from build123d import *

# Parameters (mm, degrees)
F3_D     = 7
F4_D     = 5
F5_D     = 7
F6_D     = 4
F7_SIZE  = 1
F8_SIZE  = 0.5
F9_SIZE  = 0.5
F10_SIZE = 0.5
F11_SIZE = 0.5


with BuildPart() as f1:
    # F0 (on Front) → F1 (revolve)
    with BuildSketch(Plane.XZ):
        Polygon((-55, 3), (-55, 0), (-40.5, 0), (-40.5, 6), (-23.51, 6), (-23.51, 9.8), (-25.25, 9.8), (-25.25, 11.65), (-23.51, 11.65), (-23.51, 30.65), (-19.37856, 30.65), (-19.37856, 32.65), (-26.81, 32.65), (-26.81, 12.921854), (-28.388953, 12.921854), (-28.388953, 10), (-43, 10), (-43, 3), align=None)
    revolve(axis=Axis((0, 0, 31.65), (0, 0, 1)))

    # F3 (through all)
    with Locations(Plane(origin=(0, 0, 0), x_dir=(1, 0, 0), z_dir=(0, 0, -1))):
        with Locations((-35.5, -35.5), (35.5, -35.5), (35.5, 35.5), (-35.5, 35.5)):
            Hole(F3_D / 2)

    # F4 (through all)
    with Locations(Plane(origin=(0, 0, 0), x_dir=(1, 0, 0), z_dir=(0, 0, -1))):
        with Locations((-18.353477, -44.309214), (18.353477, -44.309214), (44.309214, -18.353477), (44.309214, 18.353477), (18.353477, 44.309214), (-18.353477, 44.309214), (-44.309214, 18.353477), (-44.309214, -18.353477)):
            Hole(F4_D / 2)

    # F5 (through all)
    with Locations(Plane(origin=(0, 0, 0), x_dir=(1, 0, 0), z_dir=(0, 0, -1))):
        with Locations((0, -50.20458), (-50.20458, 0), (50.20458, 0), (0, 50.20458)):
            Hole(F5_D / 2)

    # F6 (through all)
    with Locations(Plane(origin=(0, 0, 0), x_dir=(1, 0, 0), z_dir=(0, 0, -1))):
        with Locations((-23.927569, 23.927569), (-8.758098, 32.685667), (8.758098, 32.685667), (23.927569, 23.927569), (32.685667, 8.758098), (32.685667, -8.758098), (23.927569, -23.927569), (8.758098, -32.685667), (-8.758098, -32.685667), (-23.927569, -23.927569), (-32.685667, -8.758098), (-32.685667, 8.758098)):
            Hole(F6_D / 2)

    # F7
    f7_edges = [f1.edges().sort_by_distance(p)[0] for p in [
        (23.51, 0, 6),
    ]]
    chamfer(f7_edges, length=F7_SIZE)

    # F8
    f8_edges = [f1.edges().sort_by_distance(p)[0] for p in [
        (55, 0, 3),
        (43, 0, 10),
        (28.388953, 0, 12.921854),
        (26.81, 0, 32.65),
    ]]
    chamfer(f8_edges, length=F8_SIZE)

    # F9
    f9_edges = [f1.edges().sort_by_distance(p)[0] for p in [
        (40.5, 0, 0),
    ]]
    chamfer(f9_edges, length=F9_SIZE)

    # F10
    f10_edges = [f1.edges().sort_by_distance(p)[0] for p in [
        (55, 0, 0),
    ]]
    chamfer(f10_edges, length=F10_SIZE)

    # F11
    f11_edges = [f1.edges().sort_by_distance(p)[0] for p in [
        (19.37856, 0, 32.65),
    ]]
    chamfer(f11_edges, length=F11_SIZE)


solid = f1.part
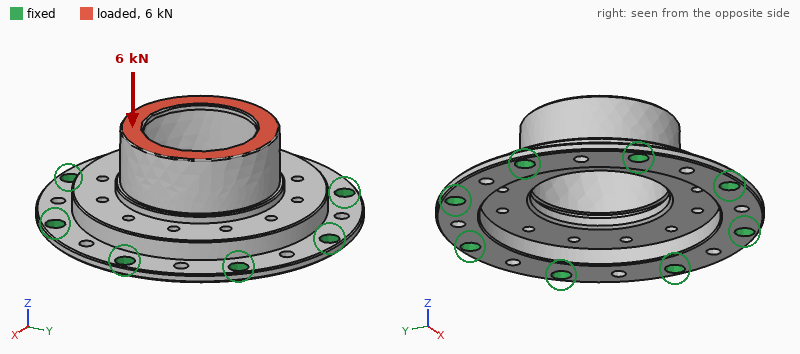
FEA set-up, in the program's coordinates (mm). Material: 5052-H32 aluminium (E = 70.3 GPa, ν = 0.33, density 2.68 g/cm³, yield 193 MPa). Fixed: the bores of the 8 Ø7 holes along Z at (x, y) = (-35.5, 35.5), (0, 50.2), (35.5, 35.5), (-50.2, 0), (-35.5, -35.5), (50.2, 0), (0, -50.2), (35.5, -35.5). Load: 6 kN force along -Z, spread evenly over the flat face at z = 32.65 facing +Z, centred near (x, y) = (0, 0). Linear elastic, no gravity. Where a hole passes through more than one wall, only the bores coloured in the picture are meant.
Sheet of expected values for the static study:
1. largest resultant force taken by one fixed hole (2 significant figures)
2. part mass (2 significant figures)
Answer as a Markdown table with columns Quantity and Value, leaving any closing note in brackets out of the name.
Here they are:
| Quantity | Value |
|---|---|
| largest resultant force taken by one fixed hole | 1.4 kN |
| part mass | 110 g |
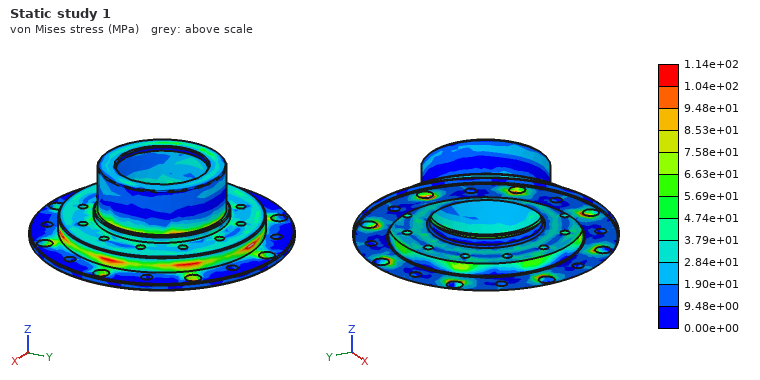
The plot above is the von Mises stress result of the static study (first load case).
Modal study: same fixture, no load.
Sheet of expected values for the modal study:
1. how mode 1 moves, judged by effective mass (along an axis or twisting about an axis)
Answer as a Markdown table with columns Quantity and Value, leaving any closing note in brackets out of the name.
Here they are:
| Quantity | Value |
|---|---|
| how mode 1 moves, judged by effective mass | along Z |
